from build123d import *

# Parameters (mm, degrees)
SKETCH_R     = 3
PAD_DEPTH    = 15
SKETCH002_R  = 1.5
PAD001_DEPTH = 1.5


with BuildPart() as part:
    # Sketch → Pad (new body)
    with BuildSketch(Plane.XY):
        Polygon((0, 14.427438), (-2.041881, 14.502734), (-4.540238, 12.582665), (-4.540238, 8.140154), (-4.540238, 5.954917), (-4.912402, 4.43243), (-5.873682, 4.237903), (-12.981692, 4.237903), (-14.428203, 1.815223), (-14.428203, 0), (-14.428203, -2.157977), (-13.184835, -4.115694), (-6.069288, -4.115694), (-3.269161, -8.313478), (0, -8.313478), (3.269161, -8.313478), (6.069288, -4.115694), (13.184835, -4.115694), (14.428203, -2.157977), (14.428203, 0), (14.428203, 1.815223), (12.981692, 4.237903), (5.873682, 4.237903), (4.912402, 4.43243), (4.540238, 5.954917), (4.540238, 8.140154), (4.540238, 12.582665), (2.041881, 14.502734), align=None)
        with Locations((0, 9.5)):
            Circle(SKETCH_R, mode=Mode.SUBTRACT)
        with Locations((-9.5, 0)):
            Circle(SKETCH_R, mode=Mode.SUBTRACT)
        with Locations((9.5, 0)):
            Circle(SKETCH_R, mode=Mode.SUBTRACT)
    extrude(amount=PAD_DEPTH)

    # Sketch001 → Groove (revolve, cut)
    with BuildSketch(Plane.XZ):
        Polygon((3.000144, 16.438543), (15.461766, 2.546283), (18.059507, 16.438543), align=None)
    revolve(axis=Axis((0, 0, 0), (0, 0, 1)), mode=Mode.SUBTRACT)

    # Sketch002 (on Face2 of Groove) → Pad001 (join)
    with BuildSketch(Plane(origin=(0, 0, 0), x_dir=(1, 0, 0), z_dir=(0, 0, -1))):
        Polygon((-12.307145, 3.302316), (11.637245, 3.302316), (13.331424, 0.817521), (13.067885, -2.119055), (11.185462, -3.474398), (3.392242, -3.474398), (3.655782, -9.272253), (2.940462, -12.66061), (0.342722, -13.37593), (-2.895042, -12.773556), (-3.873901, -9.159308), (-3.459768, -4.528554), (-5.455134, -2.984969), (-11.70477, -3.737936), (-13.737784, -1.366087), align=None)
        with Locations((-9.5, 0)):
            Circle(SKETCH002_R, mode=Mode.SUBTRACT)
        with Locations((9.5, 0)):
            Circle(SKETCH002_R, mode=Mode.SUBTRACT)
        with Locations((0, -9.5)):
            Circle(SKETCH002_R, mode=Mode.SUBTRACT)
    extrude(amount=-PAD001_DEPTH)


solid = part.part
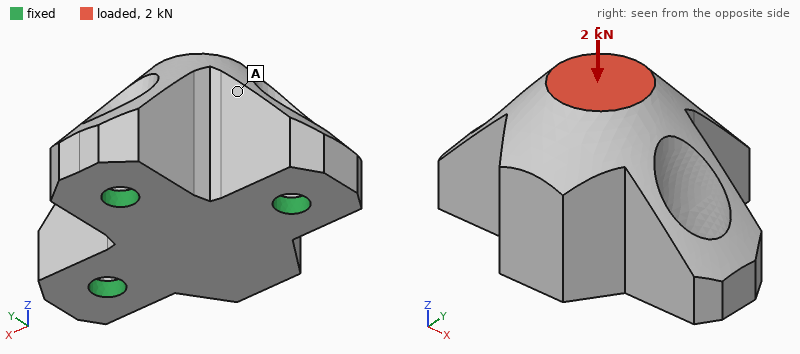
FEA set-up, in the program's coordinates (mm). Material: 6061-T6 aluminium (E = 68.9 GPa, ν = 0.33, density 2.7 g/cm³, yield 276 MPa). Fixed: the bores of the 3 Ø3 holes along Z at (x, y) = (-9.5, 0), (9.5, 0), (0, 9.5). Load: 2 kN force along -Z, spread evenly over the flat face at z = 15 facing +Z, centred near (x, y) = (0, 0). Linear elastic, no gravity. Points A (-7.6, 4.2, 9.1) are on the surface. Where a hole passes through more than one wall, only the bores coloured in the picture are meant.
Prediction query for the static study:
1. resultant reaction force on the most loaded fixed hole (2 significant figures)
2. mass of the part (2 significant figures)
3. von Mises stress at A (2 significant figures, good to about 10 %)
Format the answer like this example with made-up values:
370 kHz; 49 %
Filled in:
1000 N; 8.6 g; 34 MPa
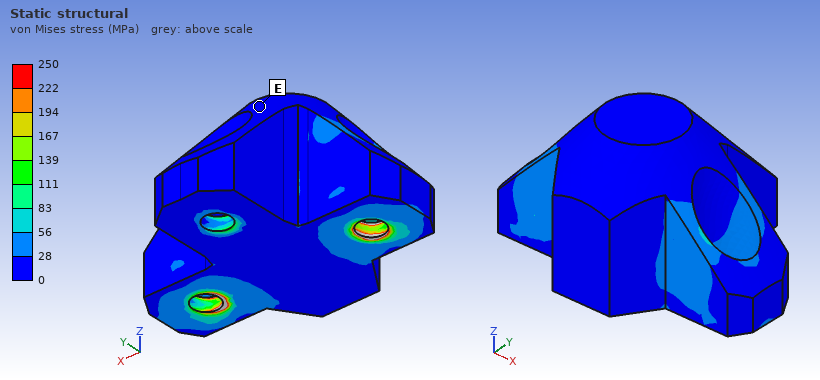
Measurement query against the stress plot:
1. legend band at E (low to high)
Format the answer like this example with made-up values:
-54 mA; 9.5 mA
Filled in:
0 to 28 MPa
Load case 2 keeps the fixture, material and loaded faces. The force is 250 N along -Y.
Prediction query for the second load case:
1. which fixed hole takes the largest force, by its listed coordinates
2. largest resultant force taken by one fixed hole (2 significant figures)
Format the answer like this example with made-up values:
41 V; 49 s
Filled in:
(0, 9.5); 360 N
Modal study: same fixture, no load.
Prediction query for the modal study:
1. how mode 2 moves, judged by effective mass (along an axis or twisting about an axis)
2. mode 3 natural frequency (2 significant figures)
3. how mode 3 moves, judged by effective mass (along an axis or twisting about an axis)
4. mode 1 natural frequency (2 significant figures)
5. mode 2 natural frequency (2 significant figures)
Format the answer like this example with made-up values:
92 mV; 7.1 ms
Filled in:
along X; 32 kHz; along Z; 15 kHz; 25 kHz
